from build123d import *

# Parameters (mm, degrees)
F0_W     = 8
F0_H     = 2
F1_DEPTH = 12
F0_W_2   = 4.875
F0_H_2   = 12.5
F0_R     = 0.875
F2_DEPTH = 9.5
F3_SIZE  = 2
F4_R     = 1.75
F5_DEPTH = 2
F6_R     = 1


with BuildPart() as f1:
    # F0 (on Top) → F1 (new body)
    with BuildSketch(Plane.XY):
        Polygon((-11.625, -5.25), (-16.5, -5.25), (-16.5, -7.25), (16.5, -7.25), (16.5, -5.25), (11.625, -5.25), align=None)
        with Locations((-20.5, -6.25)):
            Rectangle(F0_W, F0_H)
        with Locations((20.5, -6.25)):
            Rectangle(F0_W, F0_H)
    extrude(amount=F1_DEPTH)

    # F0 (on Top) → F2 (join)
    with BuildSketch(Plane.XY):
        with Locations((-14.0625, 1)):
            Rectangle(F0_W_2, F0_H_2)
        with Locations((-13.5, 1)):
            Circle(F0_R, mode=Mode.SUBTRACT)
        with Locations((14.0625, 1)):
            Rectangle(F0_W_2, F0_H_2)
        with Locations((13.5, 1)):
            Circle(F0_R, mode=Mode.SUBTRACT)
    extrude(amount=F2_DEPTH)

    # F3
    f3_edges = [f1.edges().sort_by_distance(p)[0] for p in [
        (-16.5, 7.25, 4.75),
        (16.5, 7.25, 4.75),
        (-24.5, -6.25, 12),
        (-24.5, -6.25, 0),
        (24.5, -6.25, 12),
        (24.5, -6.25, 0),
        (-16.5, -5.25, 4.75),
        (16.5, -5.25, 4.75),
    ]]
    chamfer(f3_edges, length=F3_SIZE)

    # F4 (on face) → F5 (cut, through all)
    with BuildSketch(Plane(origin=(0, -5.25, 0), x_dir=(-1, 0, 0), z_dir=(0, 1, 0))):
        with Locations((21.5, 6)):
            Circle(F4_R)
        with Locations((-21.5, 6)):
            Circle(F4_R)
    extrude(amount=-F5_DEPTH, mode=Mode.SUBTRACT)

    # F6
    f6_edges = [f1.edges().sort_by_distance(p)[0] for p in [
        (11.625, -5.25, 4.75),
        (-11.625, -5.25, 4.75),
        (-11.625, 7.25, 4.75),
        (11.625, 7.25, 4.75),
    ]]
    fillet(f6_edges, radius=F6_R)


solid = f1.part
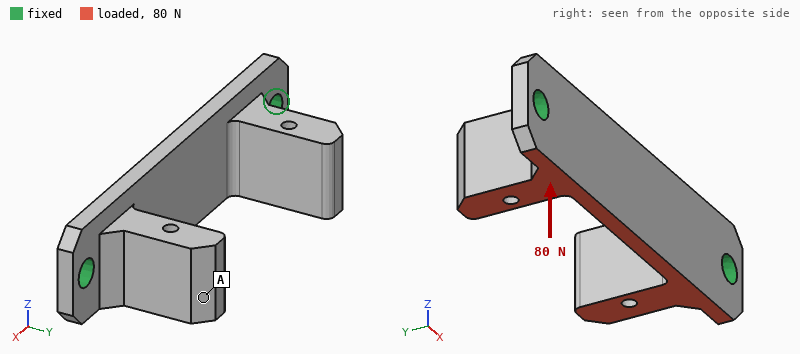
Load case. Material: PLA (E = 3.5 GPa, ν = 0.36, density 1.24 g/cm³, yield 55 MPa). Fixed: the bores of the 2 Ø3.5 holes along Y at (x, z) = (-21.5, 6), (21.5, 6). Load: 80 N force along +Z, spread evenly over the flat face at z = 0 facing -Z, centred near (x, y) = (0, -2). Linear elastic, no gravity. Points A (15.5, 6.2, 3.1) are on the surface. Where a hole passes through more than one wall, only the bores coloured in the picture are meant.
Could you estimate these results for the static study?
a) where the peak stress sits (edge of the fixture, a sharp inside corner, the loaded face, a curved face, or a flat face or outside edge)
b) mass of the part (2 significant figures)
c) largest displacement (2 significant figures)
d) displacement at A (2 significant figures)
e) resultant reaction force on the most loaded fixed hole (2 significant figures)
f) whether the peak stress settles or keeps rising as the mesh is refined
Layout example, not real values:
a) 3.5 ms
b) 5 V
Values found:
a) edge of the fixture
b) 2.8 g
c) 0.16 mm
d) 0.13 mm
e) 40 N
f) keeps rising
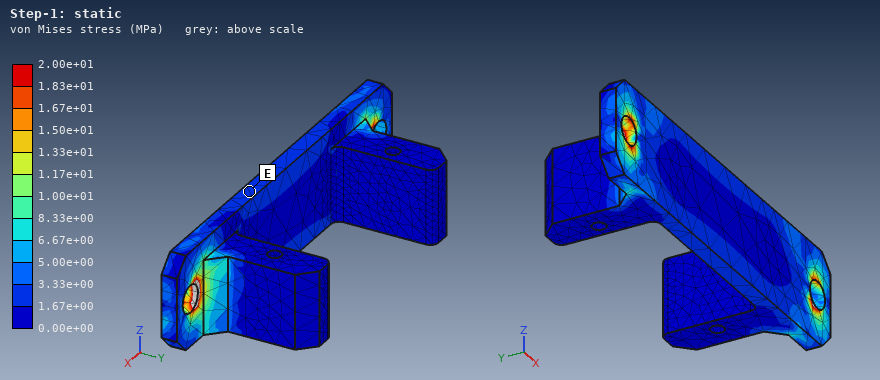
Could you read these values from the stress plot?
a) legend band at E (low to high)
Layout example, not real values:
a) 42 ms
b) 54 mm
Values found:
a) 1.67e+00 to 3.33e+00 MPa
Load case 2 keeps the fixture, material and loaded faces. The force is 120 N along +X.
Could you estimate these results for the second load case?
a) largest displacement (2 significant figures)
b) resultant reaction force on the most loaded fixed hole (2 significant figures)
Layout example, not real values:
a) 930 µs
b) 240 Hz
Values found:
a) 0.18 mm
b) 62 N
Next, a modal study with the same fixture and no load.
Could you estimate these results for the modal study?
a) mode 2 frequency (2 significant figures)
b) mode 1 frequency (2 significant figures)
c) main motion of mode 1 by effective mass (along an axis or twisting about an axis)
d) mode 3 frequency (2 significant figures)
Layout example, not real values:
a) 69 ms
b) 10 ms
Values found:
a) 2700 Hz
b) 1500 Hz
c) along Y
d) 2800 Hz
